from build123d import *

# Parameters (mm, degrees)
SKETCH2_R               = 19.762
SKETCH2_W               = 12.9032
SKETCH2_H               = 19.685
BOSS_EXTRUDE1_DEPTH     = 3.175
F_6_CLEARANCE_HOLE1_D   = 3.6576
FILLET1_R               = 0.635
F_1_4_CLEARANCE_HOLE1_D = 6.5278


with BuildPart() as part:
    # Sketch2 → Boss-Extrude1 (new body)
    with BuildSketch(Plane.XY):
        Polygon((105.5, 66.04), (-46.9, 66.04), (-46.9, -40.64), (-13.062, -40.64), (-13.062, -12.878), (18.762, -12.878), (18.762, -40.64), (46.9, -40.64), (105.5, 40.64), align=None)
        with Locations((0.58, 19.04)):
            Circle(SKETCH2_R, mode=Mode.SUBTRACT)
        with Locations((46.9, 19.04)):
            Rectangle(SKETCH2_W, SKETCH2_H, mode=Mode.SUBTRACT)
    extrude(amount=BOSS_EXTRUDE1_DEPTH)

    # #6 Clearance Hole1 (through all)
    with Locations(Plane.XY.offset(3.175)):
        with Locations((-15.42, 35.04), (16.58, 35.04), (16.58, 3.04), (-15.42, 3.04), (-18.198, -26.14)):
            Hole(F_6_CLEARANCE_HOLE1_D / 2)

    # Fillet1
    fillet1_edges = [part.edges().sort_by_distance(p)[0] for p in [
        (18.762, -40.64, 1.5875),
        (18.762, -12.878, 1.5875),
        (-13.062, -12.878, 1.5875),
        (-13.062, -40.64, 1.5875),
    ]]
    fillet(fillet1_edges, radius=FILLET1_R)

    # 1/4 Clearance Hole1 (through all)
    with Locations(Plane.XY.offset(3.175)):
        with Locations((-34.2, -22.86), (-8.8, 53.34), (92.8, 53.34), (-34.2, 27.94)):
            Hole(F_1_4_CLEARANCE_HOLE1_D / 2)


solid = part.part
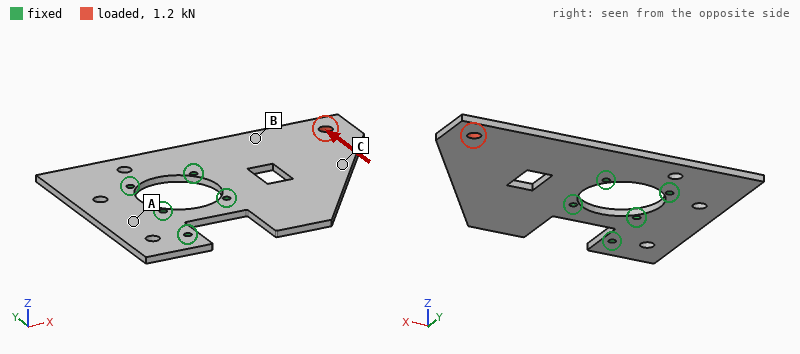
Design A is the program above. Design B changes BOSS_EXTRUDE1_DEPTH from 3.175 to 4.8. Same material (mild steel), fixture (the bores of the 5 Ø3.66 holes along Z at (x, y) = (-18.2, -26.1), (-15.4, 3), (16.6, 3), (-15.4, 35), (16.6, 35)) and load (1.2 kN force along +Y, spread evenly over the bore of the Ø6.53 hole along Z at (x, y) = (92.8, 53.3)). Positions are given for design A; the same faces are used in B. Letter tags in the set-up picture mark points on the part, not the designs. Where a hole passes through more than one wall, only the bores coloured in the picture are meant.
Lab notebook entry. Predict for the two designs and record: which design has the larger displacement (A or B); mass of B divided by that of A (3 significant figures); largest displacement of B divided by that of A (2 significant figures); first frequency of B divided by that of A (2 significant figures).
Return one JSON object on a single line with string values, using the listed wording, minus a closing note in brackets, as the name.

{"which design has the larger displacement": "A", "mass of B divided by that of A": "1.51", "largest displacement of B divided by that of A": "0.66", "first frequency of B divided by that of A": "1.5"}
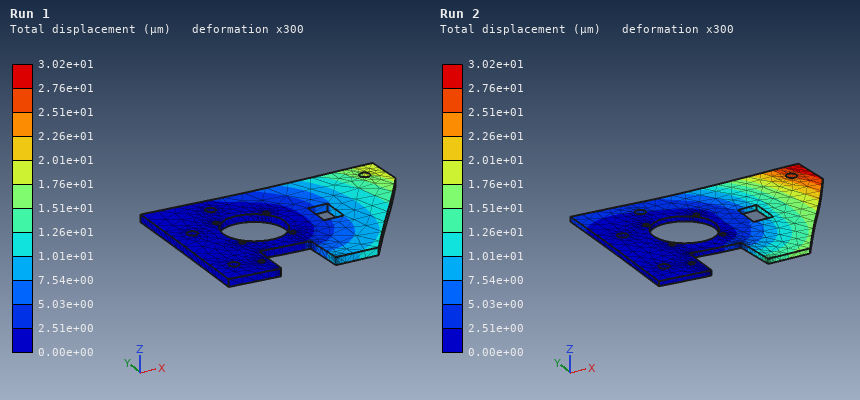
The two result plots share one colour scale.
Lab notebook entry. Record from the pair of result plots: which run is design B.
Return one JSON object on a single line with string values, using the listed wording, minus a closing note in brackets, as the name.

{"which run is design B": "Run 1"}
